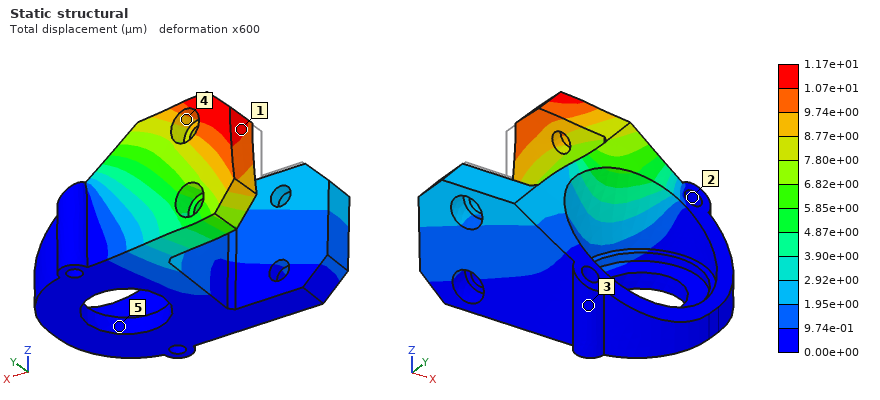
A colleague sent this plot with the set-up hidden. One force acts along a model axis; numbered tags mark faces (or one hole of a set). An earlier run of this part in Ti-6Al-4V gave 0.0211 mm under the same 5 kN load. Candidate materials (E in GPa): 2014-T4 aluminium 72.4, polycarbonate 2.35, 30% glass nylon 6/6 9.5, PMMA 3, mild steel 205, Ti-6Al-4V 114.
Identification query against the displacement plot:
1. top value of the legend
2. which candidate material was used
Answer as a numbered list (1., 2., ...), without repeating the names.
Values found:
1. 1.17e+01 µm
2. mild steel
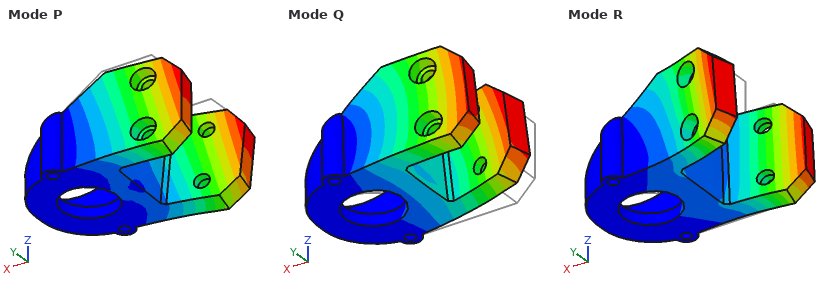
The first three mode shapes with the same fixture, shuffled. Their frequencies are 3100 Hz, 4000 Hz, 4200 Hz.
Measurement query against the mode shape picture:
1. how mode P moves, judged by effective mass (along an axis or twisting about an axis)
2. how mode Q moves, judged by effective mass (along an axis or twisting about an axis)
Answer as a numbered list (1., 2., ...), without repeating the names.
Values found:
1. along Y
2. along Z
